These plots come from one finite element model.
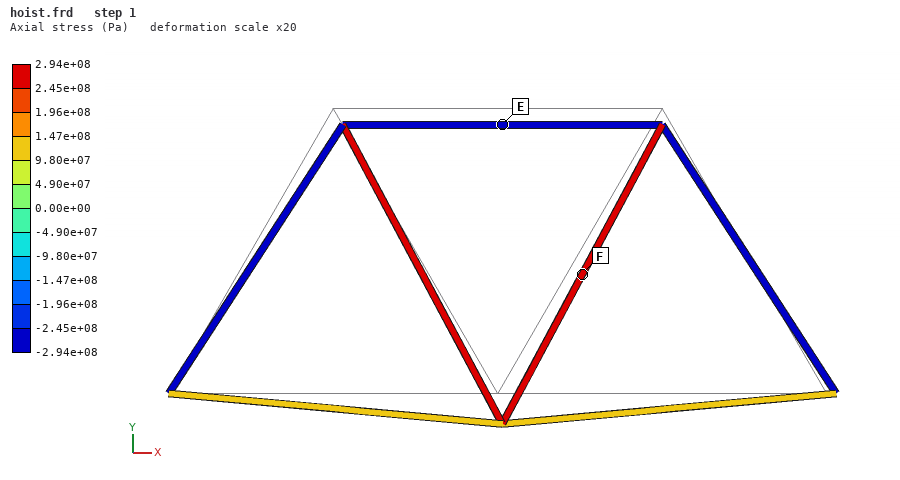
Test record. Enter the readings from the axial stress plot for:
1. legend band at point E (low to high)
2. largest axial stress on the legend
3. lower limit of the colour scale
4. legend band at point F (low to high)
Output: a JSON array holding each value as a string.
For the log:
["-2.94e+08 to -2.45e+08 Pa", "2.94e+08 Pa", "-2.94e+08 Pa", "2.45e+08 to 2.94e+08 Pa"]
